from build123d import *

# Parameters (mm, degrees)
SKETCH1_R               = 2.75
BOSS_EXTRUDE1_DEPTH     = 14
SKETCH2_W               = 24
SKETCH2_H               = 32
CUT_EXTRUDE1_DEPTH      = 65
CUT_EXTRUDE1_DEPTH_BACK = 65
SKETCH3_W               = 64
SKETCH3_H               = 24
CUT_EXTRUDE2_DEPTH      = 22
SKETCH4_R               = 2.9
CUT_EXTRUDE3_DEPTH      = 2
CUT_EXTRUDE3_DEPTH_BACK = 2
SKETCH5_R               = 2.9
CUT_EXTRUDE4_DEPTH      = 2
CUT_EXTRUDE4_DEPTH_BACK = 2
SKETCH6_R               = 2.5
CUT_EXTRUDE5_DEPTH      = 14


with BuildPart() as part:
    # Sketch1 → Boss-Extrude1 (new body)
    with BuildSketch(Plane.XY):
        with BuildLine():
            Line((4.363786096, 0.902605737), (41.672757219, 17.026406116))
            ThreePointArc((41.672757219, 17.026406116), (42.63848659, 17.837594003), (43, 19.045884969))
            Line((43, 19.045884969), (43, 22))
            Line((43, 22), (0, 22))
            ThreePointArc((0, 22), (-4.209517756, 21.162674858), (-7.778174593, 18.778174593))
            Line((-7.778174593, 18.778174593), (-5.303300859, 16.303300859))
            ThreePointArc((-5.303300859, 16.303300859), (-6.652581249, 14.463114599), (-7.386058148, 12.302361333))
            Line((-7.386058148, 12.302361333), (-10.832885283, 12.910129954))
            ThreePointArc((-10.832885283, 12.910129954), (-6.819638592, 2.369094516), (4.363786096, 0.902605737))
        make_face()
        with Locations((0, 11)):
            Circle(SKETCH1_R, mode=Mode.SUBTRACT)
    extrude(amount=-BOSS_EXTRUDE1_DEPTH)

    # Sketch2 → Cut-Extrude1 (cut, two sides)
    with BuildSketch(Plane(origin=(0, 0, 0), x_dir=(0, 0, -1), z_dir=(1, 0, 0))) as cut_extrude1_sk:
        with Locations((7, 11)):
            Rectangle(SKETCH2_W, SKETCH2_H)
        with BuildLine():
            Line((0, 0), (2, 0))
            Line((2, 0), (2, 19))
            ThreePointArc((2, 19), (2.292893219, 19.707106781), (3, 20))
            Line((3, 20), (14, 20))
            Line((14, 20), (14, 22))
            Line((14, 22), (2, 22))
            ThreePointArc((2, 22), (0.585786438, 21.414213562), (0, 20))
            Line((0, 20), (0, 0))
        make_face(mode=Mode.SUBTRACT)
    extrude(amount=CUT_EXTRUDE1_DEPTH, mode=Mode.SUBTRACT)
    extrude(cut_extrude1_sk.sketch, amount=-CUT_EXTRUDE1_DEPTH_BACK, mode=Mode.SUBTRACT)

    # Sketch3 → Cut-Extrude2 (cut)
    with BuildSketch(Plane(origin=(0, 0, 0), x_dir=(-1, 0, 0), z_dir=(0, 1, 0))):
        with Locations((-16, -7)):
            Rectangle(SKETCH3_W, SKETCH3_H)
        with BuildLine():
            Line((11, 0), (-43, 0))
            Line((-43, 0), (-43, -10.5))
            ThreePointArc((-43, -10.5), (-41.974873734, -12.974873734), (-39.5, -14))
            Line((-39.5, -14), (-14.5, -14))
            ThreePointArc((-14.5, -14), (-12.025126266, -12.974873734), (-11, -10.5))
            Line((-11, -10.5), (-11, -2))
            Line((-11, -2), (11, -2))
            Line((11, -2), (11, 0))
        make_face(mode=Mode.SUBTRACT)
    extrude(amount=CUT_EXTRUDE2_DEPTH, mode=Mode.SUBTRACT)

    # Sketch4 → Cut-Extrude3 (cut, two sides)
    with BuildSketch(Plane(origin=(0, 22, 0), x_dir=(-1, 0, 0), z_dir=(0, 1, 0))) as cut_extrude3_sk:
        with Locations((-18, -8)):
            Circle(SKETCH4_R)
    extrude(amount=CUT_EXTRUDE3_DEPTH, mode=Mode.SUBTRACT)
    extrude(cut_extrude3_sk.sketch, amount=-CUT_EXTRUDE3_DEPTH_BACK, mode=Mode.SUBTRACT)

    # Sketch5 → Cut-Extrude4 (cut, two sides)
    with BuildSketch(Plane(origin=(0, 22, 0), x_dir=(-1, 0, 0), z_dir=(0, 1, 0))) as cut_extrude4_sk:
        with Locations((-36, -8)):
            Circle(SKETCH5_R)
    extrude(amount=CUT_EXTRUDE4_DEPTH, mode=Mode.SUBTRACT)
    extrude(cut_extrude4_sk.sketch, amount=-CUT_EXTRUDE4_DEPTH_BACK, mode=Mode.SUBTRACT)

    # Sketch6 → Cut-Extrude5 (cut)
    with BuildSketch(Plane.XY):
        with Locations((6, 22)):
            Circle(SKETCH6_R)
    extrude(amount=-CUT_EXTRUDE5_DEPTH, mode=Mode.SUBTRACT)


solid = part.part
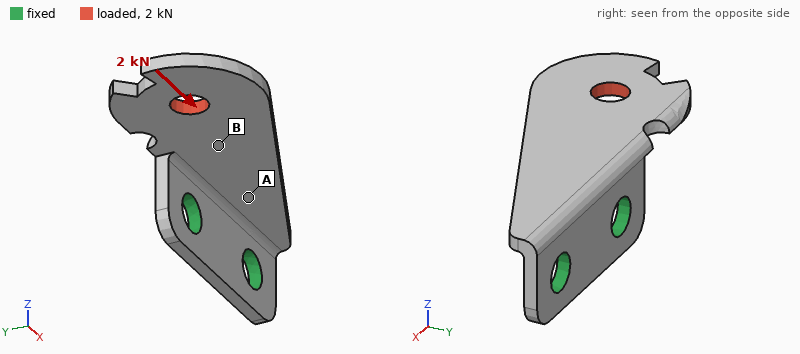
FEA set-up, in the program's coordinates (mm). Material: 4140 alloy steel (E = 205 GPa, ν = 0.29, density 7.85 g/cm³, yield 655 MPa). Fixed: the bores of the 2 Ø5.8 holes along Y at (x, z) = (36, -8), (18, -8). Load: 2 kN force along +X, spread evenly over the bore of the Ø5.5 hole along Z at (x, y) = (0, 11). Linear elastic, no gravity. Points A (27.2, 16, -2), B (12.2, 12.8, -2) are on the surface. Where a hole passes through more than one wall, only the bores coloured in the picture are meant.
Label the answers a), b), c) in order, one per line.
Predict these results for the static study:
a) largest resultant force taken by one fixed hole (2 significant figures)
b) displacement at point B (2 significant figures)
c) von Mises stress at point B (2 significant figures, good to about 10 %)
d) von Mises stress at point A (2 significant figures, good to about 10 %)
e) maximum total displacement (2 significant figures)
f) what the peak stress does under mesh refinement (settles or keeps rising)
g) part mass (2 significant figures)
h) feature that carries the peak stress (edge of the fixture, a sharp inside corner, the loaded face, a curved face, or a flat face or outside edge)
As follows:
a) 1.6 kN
b) 0.053 mm
c) 85 MPa
d) 180 MPa
e) 0.15 mm
f) keeps rising
g) 16 g
h) edge of the fixture
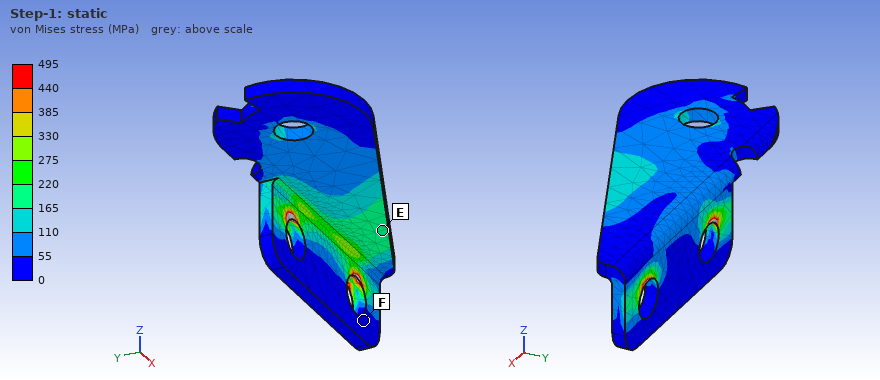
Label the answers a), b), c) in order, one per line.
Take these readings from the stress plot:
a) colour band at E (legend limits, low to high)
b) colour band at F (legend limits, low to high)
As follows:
a) 165 to 220 MPa
b) 0 to 55 MPa
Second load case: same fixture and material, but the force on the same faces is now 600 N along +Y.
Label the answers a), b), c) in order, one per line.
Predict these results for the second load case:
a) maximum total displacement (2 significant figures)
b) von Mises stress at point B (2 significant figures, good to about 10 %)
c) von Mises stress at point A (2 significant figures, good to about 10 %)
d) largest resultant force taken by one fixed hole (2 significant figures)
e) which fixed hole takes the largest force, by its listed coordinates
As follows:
a) 0.17 mm
b) 44 MPa
c) 120 MPa
d) 1.1 kN
e) (18, -8)
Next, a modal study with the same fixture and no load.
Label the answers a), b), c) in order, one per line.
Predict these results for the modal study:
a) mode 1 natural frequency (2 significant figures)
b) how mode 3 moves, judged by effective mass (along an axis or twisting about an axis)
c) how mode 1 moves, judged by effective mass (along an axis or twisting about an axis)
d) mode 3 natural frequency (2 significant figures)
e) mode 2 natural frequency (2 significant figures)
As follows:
a) 1800 Hz
b) along Y
c) along Z
d) 6100 Hz
e) 4700 Hz
